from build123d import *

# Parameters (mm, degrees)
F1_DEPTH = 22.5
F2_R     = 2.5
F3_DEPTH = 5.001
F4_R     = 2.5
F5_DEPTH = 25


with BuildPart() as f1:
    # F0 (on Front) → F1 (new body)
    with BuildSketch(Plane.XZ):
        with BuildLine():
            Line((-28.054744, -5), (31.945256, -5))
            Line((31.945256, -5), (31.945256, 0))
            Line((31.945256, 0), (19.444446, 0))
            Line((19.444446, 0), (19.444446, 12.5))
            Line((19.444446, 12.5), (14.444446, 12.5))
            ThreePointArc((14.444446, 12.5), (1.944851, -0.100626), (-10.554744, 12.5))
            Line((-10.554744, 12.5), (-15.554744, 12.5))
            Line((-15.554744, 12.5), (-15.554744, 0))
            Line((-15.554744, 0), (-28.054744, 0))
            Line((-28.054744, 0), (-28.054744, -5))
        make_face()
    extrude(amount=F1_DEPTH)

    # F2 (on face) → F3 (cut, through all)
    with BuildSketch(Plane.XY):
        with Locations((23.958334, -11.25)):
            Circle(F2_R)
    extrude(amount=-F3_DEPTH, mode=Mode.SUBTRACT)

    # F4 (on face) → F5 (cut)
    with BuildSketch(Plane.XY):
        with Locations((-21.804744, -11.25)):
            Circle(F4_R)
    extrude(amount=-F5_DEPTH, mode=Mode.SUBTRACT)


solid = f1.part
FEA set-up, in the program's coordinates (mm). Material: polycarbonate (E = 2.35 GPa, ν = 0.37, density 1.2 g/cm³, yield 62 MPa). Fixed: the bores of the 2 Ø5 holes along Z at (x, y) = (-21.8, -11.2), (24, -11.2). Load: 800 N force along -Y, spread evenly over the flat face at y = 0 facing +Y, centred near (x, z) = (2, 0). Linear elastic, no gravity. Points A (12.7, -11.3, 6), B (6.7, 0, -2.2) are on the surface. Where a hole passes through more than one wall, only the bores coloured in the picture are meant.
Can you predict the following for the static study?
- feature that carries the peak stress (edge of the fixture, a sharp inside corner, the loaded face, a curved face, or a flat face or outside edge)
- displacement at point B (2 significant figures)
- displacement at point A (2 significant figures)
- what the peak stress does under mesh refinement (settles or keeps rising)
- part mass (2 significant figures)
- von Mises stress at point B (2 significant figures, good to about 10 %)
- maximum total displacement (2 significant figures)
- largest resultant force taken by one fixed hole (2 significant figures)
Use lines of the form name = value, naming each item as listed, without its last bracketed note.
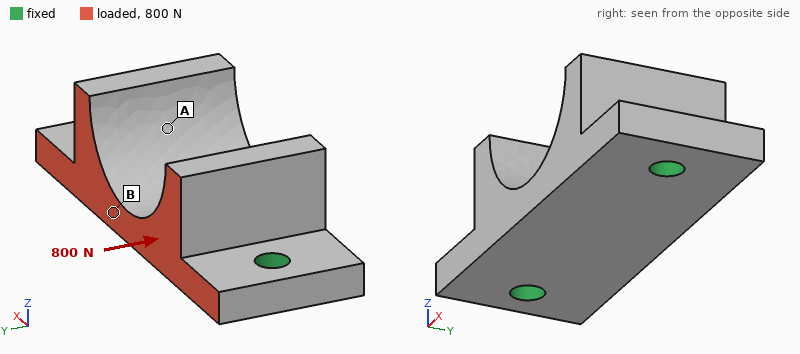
feature that carries the peak stress = edge of the fixture
displacement at point B = 0.11 mm
displacement at point A = 0.12 mm
what the peak stress does under mesh refinement = keeps rising
part mass = 13 g
von Mises stress at point B = 4.7 MPa
maximum total displacement = 0.22 mm
largest resultant force taken by one fixed hole = 420 N
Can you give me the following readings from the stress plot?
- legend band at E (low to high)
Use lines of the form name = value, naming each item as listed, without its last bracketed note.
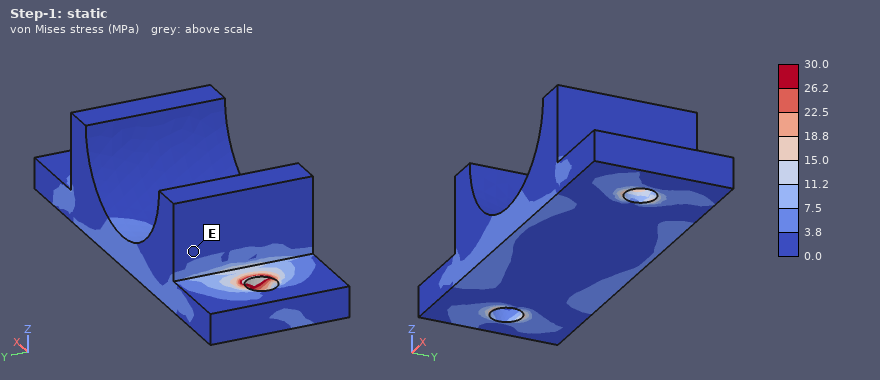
legend band at E = 0.0 to 3.8 MPa
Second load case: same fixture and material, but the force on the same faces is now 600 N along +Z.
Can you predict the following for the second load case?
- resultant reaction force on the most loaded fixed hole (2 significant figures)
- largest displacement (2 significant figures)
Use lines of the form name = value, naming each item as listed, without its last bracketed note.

resultant reaction force on the most loaded fixed hole = 320 N
largest displacement = 0.56 mm
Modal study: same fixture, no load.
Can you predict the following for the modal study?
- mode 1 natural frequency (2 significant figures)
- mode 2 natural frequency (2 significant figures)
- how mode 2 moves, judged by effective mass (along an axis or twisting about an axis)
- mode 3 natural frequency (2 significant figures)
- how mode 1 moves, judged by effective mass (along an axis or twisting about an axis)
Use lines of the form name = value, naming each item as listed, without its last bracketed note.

mode 1 natural frequency = 2500 Hz
mode 2 natural frequency = 2800 Hz
how mode 2 moves, judged by effective mass = along Y
mode 3 natural frequency = 4500 Hz
how mode 1 moves, judged by effective mass = along Z
